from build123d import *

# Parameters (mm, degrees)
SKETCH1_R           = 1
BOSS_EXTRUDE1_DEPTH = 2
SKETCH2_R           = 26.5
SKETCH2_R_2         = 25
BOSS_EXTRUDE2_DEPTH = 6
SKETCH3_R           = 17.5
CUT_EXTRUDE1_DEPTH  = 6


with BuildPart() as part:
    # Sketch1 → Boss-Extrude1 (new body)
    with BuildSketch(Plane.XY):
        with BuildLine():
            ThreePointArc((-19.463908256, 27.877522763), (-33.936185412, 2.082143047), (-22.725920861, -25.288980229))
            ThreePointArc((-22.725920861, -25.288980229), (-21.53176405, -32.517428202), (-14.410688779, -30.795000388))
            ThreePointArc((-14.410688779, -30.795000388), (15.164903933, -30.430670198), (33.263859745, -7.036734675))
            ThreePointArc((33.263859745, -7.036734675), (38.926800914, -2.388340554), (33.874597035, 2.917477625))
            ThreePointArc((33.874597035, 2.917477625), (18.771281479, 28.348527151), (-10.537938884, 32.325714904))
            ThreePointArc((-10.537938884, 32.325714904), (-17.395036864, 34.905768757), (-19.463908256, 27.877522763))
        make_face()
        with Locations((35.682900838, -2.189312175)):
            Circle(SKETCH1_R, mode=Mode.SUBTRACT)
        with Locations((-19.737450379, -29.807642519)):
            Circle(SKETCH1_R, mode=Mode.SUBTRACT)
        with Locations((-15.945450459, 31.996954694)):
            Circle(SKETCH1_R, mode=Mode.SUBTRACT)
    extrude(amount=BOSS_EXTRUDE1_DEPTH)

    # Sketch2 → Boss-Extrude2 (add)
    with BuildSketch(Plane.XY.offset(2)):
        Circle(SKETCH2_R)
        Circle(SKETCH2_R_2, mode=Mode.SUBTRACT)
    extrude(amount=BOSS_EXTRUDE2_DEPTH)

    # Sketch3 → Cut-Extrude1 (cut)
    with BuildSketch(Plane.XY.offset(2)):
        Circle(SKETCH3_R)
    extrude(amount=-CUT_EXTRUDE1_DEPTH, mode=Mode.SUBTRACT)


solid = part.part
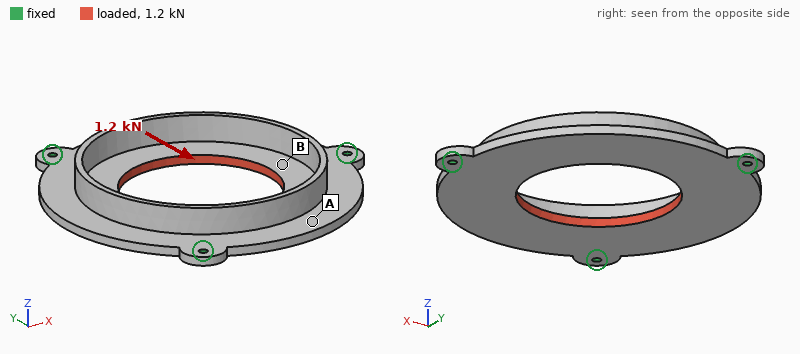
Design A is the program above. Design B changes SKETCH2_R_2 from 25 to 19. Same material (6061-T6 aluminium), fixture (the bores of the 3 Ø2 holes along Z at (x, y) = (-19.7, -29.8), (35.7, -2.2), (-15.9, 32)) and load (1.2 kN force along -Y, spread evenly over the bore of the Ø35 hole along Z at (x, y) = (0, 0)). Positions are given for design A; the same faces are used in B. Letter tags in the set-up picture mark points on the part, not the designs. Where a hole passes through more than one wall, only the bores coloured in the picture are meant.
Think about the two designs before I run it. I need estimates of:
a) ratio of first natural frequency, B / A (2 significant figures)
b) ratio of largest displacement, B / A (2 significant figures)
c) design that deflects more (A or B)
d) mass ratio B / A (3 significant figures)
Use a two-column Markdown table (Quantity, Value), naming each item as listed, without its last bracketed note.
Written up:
| Quantity | Value |
|---|---|
| ratio of first natural frequency, B / A | 1.3 |
| ratio of largest displacement, B / A | 0.89 |
| design that deflects more | A |
| mass ratio B / A | 1.71 |
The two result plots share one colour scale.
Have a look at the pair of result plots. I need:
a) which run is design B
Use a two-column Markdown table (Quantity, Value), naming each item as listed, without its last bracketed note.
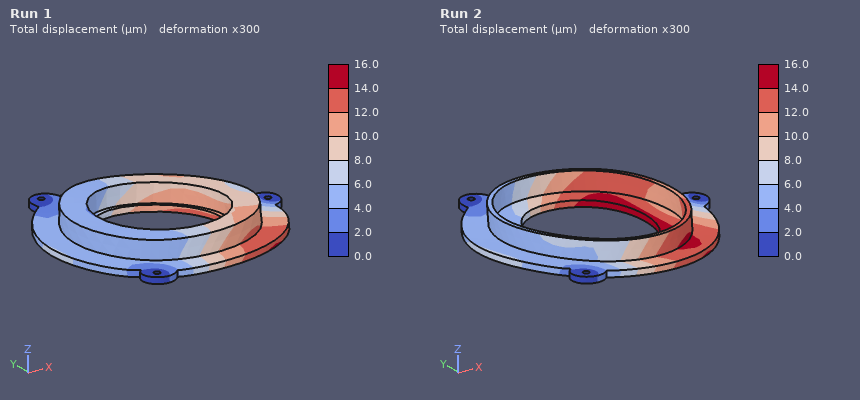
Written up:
| Quantity | Value |
|---|---|
| which run is design B | Run 1 |
